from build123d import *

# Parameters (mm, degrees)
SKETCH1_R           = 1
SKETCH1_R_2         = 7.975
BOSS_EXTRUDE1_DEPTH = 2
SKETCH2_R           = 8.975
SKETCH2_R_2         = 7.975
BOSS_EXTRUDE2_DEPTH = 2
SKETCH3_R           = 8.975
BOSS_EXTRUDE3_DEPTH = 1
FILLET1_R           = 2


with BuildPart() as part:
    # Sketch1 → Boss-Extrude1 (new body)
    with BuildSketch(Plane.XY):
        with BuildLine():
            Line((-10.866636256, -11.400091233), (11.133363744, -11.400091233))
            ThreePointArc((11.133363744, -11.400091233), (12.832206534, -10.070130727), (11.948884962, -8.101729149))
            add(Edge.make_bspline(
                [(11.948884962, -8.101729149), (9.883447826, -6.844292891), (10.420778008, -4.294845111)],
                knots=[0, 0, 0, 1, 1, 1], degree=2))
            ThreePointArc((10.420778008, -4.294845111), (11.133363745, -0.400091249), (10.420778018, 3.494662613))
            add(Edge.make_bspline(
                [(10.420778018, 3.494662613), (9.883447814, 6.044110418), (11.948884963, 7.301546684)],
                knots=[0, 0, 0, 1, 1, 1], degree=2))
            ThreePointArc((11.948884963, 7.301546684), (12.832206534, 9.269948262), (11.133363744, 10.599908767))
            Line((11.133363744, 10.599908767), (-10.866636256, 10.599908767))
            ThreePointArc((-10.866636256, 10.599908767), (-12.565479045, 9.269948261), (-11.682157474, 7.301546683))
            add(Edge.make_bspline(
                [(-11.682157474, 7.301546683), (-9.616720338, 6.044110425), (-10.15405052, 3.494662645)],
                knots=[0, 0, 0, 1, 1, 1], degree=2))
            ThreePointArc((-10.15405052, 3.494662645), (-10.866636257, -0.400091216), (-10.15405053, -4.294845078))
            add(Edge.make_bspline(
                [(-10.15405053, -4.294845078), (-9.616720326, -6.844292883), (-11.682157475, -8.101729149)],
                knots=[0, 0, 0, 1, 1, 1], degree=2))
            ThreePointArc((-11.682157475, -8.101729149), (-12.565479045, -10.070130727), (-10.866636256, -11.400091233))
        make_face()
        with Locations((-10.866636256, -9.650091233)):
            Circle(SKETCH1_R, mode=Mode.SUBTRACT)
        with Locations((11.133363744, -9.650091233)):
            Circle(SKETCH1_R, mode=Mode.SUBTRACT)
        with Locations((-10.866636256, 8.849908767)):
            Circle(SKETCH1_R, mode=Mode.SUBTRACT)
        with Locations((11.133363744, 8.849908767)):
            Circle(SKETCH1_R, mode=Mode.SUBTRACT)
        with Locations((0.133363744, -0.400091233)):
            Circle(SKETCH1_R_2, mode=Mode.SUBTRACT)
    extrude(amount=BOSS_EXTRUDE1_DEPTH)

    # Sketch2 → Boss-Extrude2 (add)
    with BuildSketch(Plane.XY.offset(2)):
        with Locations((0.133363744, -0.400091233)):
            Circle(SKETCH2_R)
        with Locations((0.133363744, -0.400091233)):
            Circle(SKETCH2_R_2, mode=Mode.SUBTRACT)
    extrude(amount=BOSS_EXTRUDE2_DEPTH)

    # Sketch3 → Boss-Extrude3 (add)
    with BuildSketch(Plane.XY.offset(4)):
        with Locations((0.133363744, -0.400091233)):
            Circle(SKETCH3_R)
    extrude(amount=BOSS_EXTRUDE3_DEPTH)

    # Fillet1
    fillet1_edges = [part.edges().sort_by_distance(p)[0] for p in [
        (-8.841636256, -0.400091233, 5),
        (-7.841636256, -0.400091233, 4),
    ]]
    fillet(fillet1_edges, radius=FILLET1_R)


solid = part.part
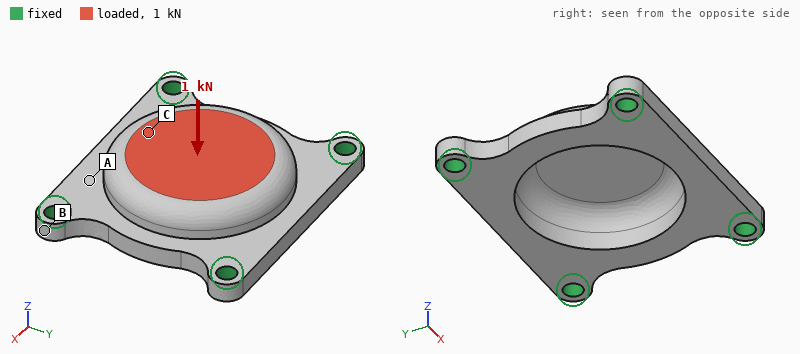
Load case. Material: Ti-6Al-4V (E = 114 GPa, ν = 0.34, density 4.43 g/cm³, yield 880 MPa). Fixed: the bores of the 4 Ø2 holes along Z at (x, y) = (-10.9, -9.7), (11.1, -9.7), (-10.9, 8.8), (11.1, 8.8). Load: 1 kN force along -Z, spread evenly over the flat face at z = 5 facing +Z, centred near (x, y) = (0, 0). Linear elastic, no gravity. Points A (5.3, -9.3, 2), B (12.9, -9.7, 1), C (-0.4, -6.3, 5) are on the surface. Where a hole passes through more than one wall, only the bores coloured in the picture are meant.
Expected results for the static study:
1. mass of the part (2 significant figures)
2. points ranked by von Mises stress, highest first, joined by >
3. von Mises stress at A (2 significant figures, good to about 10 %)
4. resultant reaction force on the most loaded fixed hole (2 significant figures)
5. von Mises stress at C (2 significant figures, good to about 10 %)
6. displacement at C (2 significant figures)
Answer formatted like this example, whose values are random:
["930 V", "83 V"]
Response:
["4.0 g", "C > A > B", "62 MPa", "360 N", "110 MPa", "23 µm"]
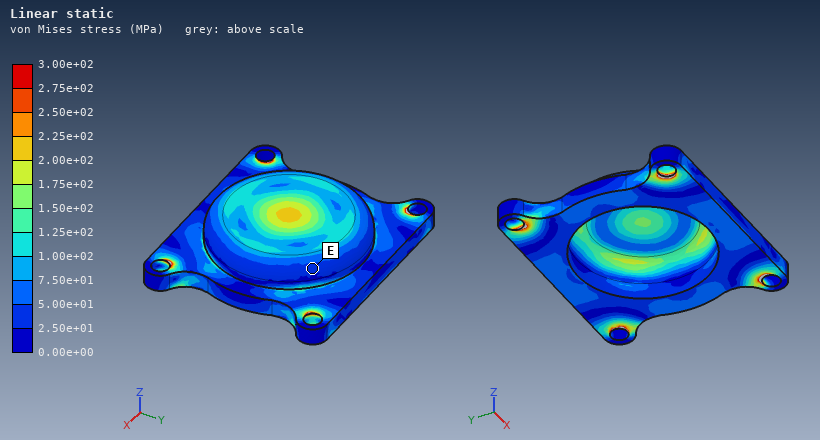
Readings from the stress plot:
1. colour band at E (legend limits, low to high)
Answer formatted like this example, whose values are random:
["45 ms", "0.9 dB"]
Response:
["2.50e+01 to 5.00e+01 MPa"]
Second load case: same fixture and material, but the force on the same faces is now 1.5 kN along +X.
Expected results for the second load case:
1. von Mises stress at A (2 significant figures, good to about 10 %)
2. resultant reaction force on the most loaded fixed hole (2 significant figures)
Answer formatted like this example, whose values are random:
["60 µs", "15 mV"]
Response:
["72 MPa", "430 N"]
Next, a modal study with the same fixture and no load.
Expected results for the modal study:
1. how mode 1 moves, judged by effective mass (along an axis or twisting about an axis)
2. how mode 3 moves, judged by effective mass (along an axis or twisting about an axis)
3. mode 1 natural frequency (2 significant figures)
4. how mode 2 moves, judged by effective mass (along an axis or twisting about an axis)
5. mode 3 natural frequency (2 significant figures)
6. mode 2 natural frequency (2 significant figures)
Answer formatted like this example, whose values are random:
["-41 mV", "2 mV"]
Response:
["along Z", "twisting about Y", "22 kHz", "twisting about X", "31 kHz", "26 kHz"]
